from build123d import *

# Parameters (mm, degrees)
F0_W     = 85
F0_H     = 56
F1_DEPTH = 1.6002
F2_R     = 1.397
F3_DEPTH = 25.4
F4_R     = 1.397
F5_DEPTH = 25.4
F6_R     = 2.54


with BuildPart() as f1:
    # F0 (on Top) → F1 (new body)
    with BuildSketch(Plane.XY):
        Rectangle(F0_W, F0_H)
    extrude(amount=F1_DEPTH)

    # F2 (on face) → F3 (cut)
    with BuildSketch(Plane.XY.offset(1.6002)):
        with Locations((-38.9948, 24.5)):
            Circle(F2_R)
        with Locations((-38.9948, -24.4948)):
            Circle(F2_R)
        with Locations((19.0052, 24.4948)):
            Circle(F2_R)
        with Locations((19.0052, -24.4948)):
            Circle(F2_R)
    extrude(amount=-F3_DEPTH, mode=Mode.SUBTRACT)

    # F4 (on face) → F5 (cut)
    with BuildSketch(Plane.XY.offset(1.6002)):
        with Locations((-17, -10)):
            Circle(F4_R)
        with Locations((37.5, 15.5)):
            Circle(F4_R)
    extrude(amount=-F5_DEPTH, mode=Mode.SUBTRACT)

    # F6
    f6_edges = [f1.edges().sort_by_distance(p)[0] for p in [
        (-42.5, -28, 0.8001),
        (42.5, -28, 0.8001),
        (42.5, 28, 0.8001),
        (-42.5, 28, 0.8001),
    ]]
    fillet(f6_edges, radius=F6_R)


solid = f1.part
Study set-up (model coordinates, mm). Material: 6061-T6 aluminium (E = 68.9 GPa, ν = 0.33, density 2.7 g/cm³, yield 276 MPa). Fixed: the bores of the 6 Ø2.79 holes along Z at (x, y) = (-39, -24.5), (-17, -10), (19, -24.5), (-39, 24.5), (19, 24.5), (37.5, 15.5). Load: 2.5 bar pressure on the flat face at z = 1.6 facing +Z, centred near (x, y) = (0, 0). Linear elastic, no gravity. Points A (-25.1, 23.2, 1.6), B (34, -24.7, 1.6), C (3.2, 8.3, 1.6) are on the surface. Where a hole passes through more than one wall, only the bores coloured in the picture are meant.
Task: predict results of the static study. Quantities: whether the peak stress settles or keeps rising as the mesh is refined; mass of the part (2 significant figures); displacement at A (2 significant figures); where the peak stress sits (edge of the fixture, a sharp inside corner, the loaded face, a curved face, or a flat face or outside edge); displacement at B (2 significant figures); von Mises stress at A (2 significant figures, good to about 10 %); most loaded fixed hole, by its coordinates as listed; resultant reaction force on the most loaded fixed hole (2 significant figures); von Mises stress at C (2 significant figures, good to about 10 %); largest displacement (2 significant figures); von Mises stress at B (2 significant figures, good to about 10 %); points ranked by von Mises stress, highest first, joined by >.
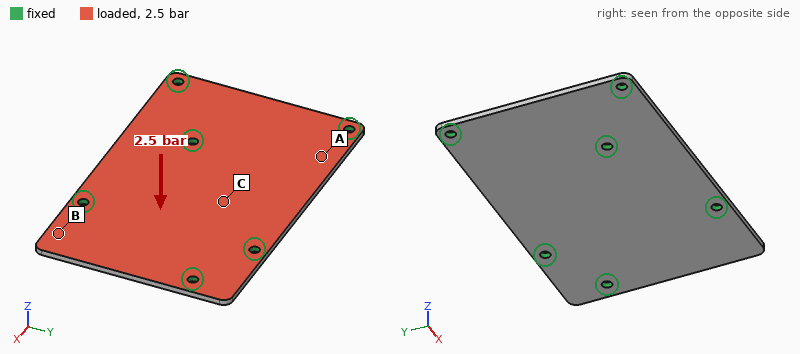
keeps rising
20 g
0.15 mm
edge of the fixture
0.15 mm
40 MPa
(-17, -10)
350 N
58 MPa
0.29 mm
19 MPa
C > A > B
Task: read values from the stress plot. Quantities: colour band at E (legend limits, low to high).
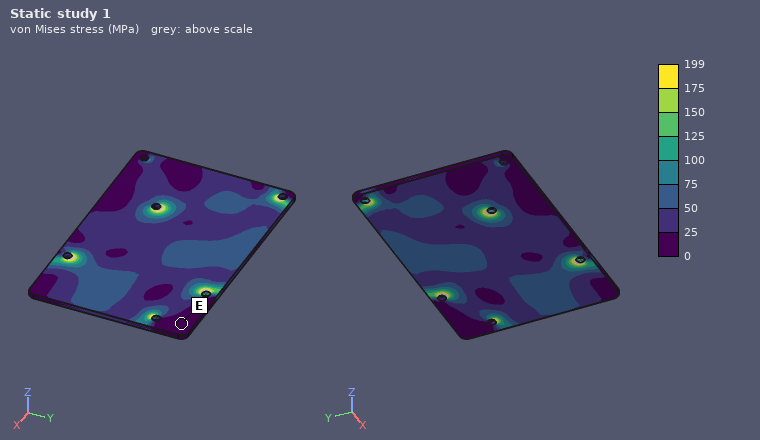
0 to 25 MPa
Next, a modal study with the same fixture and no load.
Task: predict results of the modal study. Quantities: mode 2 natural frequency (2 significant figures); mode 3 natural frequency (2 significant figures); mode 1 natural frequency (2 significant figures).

2900 Hz
4000 Hz
2800 Hz
